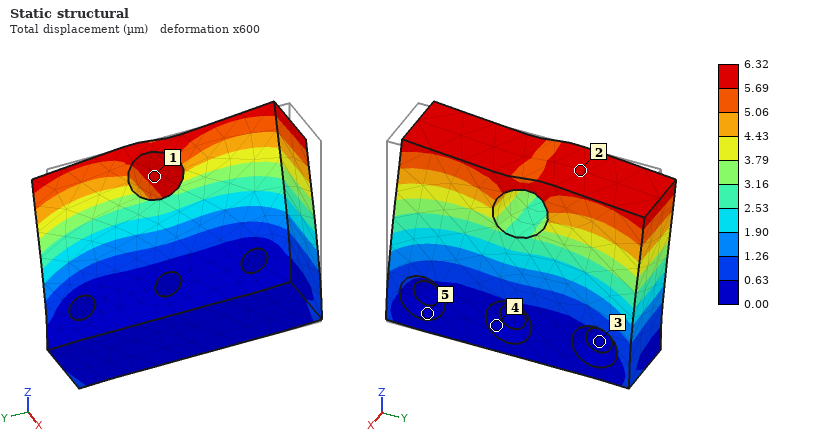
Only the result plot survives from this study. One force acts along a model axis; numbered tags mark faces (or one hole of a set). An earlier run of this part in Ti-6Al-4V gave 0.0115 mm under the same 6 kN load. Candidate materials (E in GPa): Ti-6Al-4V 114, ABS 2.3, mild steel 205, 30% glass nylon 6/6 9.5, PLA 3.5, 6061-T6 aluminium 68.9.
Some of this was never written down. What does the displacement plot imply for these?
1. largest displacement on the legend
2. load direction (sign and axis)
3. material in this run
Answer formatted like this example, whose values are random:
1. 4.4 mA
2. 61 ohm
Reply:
1. 6.32 µm
2. +Y
3. mild steel
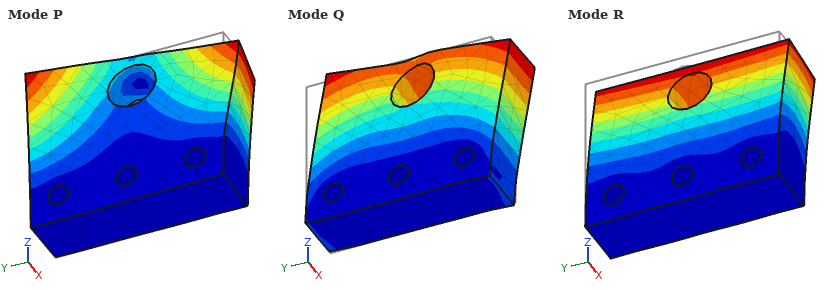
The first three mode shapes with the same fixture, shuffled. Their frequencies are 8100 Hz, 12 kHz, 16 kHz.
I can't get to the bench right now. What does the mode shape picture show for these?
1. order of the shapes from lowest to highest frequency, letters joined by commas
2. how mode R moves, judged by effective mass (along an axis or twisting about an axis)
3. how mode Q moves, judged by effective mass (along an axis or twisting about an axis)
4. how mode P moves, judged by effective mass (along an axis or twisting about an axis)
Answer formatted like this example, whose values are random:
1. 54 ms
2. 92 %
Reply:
1. R, P, Q
2. along X
3. along Y
4. twisting about Z
